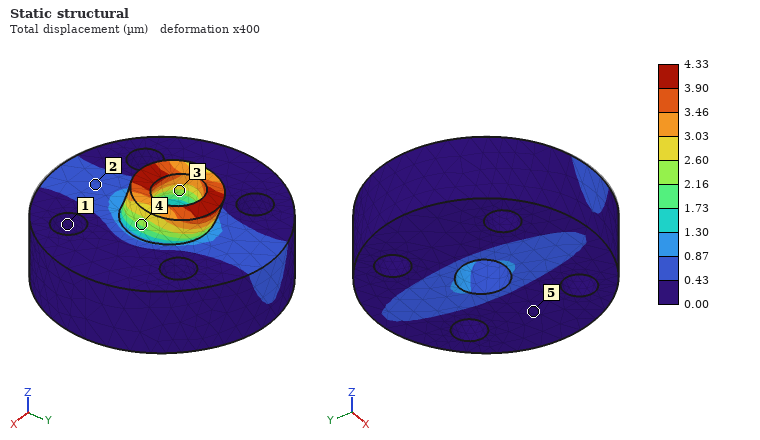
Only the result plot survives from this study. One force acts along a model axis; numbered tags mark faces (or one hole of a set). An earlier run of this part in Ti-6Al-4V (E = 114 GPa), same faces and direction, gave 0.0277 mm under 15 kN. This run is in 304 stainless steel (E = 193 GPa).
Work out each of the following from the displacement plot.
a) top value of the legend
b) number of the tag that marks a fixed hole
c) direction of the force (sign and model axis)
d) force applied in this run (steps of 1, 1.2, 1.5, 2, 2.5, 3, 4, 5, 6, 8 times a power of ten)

4.33 µm
1
+Y
4 kN
